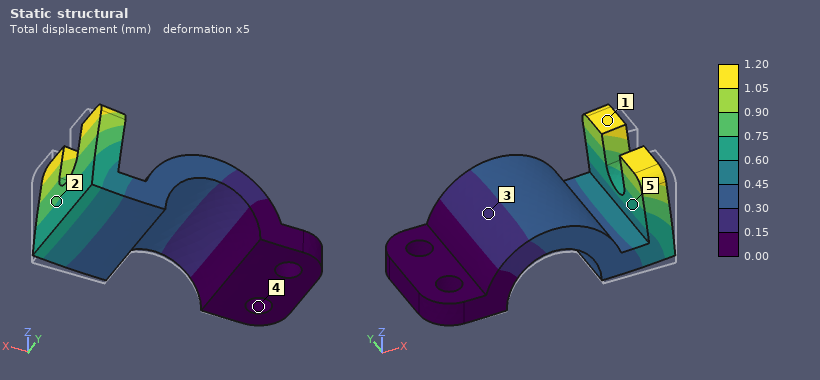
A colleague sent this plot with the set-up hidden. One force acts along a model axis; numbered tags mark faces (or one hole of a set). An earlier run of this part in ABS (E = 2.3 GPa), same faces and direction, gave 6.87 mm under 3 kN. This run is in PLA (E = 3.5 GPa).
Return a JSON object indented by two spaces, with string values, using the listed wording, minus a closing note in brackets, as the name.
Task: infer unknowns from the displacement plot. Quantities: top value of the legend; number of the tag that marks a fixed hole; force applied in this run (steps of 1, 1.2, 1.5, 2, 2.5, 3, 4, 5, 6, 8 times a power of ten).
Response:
{
  "top value of the legend": "1.20 mm",
  "number of the tag that marks a fixed hole": "4",
  "force applied in this run": "800 N"
}
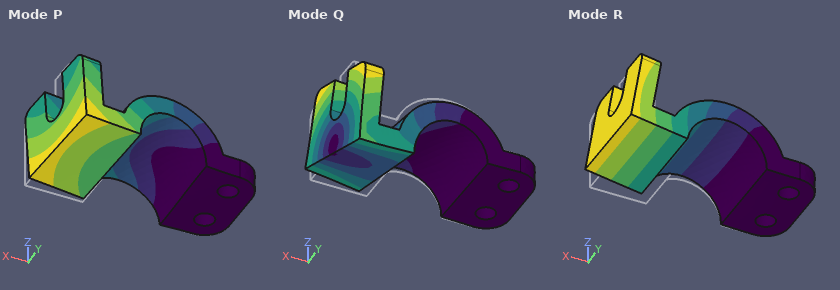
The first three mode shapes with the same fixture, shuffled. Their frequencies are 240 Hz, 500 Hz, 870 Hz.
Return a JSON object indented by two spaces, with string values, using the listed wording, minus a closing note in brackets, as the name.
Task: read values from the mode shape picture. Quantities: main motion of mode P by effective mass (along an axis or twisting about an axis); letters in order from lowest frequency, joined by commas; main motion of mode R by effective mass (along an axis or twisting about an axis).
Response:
{
  "main motion of mode P by effective mass": "along Y",
  "letters in order from lowest frequency, joined by commas": "R, P, Q",
  "main motion of mode R by effective mass": "along Z"
}
